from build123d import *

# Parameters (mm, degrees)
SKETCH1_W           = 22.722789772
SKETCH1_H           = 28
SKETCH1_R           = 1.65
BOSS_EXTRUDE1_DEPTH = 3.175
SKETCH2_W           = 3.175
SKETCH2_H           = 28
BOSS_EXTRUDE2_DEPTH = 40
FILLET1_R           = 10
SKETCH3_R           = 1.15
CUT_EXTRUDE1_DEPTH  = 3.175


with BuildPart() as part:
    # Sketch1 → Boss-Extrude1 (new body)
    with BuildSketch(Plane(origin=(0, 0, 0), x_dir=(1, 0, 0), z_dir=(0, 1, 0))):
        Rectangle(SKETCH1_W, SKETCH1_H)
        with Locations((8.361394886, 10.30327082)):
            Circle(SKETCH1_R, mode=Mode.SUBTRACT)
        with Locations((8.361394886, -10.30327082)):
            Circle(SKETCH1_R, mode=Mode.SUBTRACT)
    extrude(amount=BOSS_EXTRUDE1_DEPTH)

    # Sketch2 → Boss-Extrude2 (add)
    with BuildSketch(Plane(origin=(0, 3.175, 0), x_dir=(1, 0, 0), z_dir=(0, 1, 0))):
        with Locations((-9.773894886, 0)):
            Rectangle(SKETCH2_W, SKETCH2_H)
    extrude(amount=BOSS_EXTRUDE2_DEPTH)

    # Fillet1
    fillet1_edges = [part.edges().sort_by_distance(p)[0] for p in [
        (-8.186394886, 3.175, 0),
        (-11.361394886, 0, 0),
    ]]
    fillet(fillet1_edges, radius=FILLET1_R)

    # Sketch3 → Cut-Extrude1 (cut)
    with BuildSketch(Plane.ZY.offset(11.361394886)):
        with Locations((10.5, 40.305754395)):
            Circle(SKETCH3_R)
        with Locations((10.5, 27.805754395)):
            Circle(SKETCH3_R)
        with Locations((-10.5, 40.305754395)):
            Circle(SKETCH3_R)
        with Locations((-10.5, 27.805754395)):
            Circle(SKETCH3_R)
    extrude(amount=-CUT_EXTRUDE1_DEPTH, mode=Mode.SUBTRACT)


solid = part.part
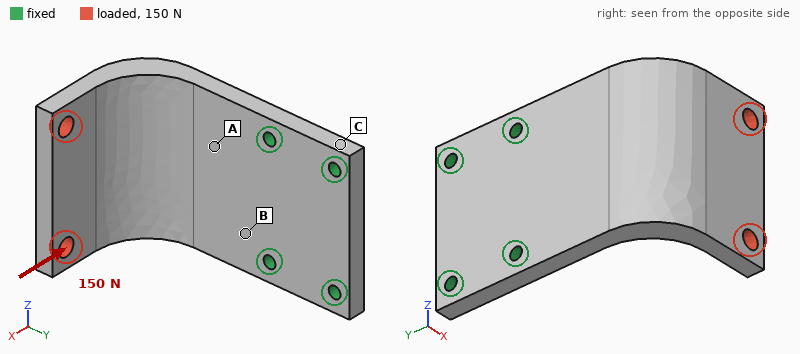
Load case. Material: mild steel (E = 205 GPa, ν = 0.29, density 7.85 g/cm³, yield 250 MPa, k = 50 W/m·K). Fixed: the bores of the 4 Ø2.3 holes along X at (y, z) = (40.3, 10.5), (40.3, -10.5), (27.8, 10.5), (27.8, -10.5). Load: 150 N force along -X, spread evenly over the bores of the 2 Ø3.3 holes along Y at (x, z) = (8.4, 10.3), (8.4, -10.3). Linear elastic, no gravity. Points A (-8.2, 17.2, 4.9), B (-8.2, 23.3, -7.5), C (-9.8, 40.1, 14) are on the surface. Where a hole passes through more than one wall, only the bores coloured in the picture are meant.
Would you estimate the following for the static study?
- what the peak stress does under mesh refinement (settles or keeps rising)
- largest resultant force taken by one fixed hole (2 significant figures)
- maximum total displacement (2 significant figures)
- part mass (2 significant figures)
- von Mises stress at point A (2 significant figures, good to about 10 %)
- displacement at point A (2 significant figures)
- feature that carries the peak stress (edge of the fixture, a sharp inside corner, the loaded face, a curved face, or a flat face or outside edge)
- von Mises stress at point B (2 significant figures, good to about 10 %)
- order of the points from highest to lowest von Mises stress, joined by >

keeps rising
130 N
96 µm
43 g
47 MPa
16 µm
edge of the fixture
64 MPa
B > A > C
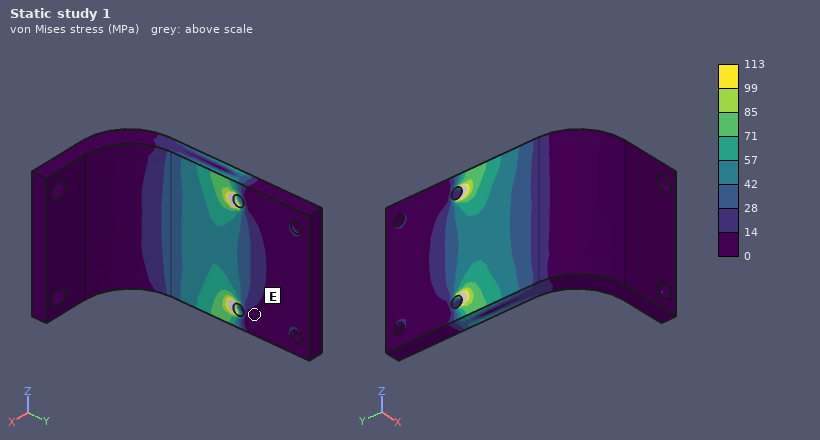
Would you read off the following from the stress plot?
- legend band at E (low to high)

0 to 14 MPa
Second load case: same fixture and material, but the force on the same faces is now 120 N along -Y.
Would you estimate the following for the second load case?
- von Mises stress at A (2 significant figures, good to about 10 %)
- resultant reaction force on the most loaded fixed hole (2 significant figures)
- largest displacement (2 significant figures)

44 MPa
59 N
86 µm
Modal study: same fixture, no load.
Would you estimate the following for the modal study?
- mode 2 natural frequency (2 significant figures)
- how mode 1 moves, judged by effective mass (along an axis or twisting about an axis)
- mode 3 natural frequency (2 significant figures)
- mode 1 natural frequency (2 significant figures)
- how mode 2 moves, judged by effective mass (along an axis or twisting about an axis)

3800 Hz
along X
6900 Hz
1600 Hz
along Z
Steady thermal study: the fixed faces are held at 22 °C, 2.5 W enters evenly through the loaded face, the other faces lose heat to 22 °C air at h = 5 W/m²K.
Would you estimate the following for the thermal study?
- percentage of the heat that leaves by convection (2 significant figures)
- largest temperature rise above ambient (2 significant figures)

6.6 %
24 K
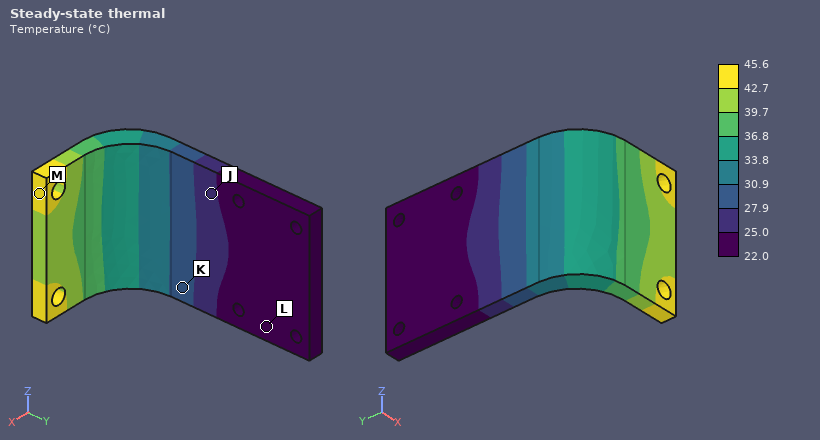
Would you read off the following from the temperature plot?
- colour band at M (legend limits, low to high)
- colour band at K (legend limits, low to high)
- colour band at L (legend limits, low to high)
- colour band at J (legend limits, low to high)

42.7 to 45.6 °C
27.9 to 30.9 °C
22.0 to 25.0 °C
25.0 to 27.9 °C
